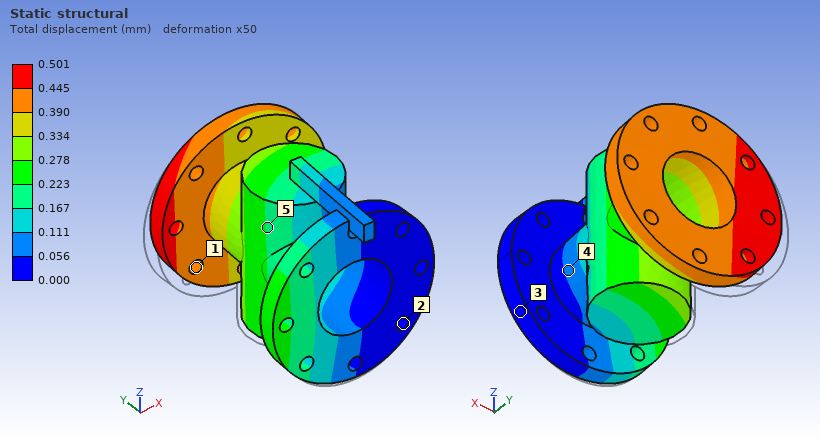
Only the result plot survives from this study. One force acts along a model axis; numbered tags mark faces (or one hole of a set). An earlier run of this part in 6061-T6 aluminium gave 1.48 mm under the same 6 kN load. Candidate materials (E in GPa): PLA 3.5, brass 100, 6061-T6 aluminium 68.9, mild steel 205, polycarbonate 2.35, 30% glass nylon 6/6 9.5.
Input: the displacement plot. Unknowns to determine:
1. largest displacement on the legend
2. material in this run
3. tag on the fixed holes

0.501 mm
mild steel
2
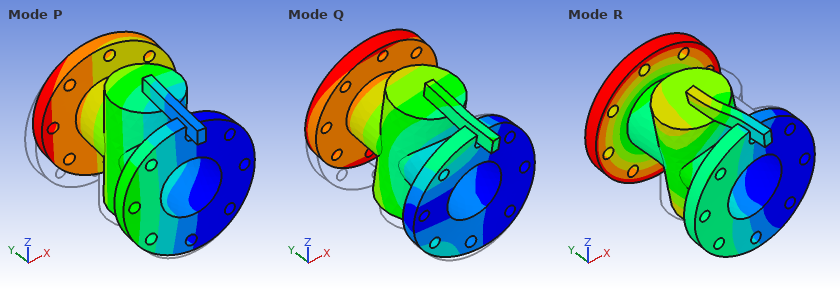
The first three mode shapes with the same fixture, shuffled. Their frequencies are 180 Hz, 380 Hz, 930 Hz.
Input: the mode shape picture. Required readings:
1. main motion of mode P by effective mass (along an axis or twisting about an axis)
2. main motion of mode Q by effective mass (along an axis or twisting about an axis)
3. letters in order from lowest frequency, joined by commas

along X
along Z
P, Q, R
